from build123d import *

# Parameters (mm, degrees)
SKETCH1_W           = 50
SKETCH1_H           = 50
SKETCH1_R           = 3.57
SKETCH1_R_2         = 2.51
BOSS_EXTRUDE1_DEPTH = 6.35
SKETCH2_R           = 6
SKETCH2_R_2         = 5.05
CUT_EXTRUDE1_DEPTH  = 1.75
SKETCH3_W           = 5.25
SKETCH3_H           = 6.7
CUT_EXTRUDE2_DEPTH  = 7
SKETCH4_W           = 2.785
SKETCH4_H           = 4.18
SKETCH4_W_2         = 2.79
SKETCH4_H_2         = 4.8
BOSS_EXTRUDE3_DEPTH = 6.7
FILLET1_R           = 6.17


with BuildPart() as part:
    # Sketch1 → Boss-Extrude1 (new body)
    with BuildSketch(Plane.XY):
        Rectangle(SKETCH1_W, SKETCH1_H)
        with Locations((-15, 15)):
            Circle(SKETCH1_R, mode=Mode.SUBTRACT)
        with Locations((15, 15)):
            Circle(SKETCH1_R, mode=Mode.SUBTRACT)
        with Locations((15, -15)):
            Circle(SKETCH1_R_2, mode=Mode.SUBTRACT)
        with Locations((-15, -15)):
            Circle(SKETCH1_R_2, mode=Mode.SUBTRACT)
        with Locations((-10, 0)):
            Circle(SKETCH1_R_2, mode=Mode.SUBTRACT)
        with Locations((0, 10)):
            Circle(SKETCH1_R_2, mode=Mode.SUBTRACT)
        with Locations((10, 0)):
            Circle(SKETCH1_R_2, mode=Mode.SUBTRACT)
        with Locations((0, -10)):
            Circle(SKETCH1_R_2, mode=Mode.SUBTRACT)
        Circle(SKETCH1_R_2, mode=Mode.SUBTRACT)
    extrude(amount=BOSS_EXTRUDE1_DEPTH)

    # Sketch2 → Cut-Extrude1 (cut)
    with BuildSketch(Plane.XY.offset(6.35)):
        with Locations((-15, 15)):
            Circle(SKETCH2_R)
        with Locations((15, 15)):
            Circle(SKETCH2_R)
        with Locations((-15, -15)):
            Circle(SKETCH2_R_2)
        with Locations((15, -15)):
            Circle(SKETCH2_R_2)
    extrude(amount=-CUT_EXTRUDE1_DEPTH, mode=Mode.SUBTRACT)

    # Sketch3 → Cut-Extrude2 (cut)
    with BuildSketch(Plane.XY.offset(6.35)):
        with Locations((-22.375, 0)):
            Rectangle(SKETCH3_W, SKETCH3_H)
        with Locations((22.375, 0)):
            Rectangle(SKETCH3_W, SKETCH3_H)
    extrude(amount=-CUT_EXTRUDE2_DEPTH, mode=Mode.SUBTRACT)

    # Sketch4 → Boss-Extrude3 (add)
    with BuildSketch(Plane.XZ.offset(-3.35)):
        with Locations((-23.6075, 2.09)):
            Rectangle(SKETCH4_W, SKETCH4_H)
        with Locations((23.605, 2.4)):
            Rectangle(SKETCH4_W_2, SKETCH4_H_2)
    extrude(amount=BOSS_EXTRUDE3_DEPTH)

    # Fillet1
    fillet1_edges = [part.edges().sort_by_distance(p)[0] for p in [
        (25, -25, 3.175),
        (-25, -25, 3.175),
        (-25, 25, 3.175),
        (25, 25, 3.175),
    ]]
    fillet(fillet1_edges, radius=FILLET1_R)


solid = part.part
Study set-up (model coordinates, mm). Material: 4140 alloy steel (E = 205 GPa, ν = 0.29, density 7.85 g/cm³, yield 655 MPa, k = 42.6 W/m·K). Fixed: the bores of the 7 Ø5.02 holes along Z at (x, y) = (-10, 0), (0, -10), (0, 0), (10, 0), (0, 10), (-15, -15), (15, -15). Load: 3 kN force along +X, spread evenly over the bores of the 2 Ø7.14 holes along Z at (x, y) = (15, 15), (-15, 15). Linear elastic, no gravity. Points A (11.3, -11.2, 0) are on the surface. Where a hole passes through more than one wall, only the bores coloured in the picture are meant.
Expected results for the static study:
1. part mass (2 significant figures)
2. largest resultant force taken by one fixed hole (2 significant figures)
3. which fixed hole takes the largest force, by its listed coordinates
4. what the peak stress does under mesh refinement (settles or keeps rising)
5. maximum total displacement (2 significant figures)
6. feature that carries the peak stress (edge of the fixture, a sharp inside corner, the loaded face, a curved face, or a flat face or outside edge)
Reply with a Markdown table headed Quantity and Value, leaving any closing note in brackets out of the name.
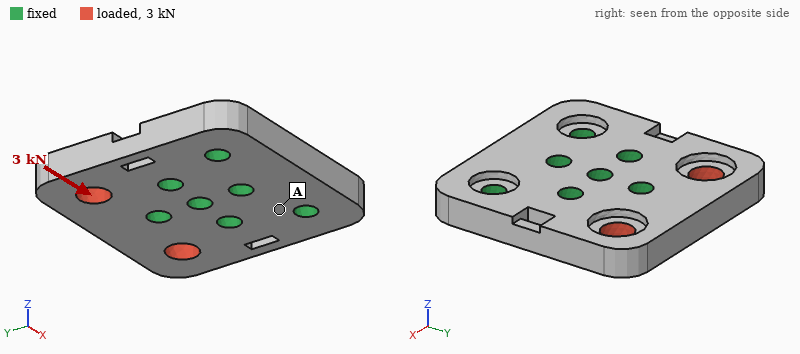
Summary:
| Quantity | Value |
|---|---|
| part mass | 110 g |
| largest resultant force taken by one fixed hole | 2.2 kN |
| which fixed hole takes the largest force, by its listed coordinates | (0, 10) |
| what the peak stress does under mesh refinement | keeps rising |
| maximum total displacement | 3.6 µm |
| feature that carries the peak stress | edge of the fixture |
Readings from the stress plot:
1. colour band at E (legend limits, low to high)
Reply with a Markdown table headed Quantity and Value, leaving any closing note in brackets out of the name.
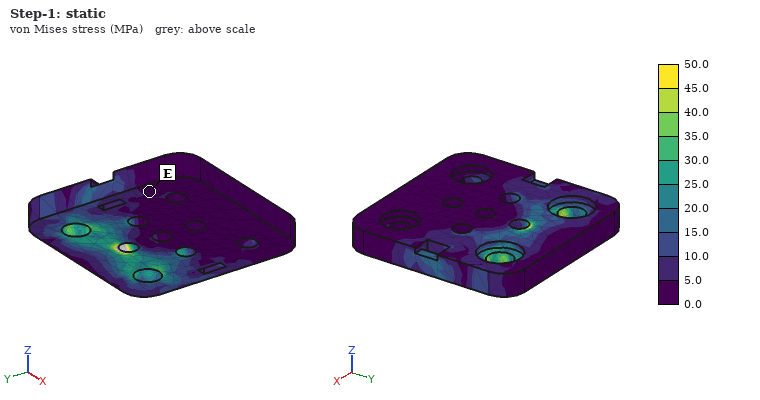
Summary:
| Quantity | Value |
|---|---|
| colour band at E | 0.0 to 5.0 MPa |
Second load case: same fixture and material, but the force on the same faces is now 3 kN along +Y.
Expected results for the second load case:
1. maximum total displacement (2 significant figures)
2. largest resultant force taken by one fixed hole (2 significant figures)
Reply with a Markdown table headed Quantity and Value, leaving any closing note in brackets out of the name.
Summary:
| Quantity | Value |
|---|---|
| maximum total displacement | 2.4 µm |
| largest resultant force taken by one fixed hole | 780 N |
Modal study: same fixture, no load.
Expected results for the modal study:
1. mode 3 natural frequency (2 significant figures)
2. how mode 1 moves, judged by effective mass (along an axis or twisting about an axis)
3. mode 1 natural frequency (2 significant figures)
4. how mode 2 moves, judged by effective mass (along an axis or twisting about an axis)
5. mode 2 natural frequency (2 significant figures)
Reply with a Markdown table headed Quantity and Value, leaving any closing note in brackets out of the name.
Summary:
| Quantity | Value |
|---|---|
| mode 3 natural frequency | 22 kHz |
| how mode 1 moves, judged by effective mass | twisting about Y |
| mode 1 natural frequency | 11 kHz |
| how mode 2 moves, judged by effective mass | along Z |
| mode 2 natural frequency | 12 kHz |
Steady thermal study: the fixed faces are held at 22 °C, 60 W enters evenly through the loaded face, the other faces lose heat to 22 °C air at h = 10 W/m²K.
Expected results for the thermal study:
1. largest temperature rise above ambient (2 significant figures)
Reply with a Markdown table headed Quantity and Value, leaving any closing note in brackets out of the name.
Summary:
| Quantity | Value |
|---|---|
| largest temperature rise above ambient | 86 K |
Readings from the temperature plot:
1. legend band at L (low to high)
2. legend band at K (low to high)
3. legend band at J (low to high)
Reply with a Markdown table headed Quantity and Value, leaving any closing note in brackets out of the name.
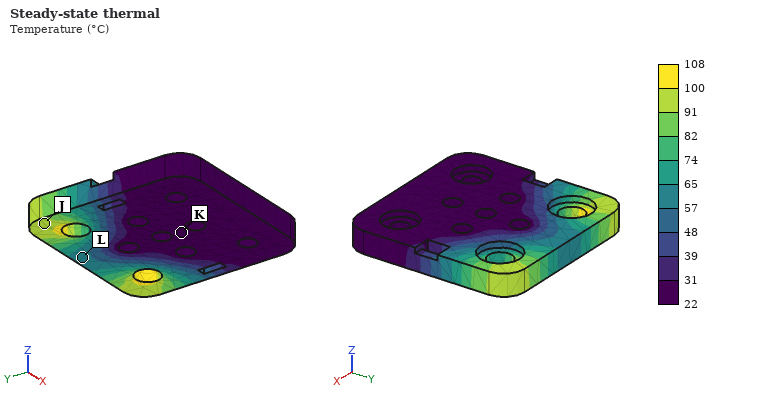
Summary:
| Quantity | Value |
|---|---|
| legend band at L | 57 to 65 °C |
| legend band at K | 22 to 31 °C |
| legend band at J | 91 to 100 °C |
